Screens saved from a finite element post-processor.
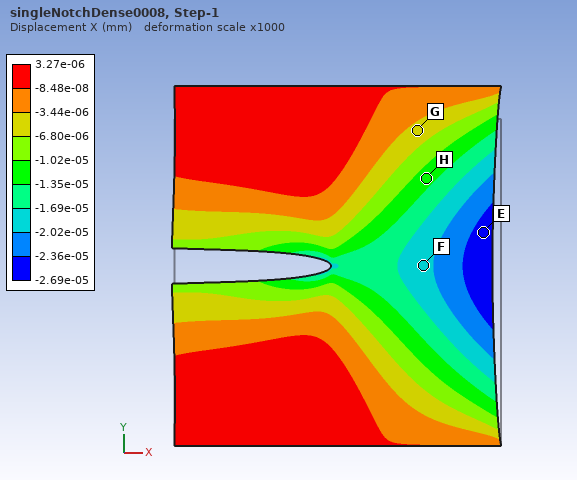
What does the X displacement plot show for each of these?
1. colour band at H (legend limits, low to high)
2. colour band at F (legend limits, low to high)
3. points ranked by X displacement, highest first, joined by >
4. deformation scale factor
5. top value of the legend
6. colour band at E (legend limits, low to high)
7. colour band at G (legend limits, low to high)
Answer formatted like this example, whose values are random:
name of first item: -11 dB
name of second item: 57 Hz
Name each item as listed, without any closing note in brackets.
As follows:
colour band at H: -1.35e-05 to -1.02e-05 mm
colour band at F: -2.02e-05 to -1.69e-05 mm
points ranked by X displacement, highest first, joined by >: G > H > F > E
deformation scale factor: 1000
top value of the legend: 3.27e-06 mm
colour band at E: -2.69e-05 to -2.36e-05 mm
colour band at G: -6.80e-06 to -3.44e-06 mm
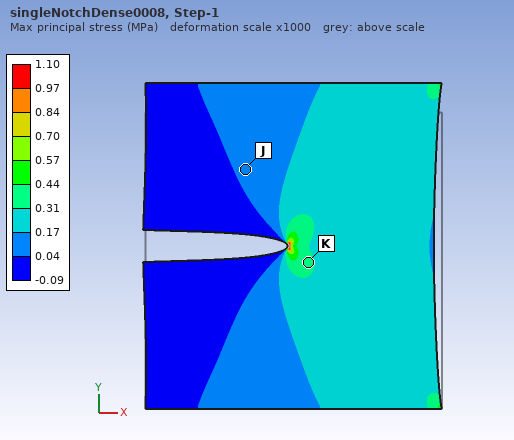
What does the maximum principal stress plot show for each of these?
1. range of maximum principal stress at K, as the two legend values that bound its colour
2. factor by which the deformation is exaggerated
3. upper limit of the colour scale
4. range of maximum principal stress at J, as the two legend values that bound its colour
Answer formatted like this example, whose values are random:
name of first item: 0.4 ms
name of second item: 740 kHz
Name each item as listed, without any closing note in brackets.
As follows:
range of maximum principal stress at K, as the two legend values that bound its colour: 0.31 to 0.44 MPa
factor by which the deformation is exaggerated: 1000
upper limit of the colour scale: 1.10 MPa
range of maximum principal stress at J, as the two legend values that bound its colour: 0.04 to 0.17 MPa
